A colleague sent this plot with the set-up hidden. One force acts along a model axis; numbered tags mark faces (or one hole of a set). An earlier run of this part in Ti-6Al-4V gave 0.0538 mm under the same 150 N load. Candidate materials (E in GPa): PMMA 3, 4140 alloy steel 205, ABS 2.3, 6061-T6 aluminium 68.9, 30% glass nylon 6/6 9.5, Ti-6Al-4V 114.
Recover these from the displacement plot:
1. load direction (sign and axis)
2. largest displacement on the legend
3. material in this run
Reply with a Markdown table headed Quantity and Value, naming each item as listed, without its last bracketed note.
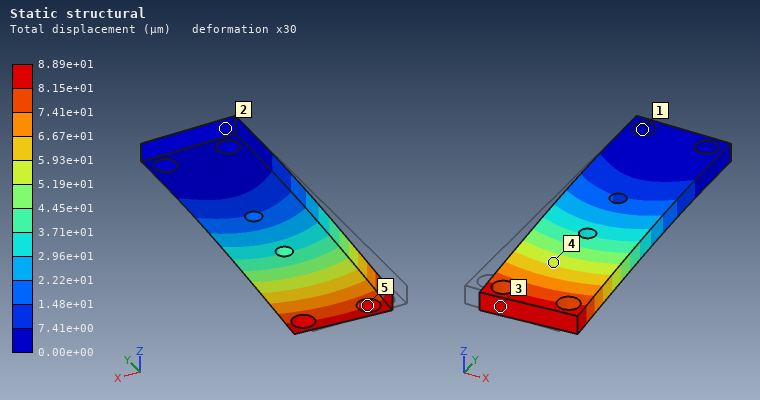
| Quantity | Value |
|---|---|
| load direction | +X |
| largest displacement on the legend | 8.89e+01 µm |
| material in this run | 6061-T6 aluminium |
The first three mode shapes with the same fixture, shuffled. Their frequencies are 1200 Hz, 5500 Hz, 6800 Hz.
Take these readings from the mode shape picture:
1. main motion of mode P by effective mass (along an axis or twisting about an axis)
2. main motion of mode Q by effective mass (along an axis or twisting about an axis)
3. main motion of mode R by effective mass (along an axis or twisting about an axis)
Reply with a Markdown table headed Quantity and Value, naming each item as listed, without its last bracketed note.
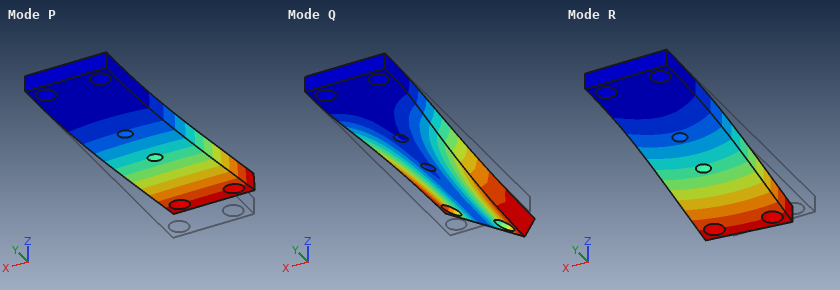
| Quantity | Value |
|---|---|
| main motion of mode P by effective mass | along Z |
| main motion of mode Q by effective mass | twisting about Y |
| main motion of mode R by effective mass | along X |
